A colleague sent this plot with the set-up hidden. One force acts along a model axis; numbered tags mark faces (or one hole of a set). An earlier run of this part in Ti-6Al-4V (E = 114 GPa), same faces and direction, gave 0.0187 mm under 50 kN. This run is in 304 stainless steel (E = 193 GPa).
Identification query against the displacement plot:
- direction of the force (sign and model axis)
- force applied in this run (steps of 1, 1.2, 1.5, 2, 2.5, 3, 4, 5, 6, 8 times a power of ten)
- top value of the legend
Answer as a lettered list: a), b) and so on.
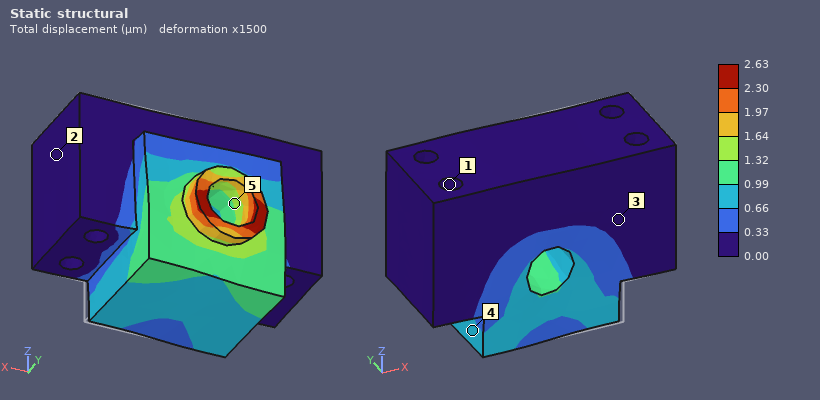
a) -X
b) 12 kN
c) 2.63 µm
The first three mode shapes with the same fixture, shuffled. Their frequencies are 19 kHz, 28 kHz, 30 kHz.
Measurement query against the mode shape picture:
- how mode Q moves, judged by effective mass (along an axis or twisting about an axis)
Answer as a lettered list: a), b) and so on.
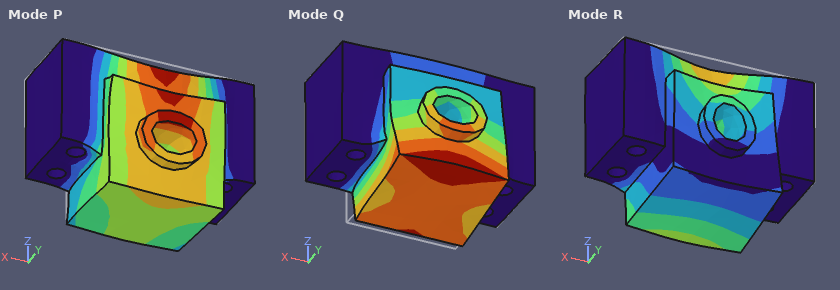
a) along Y
